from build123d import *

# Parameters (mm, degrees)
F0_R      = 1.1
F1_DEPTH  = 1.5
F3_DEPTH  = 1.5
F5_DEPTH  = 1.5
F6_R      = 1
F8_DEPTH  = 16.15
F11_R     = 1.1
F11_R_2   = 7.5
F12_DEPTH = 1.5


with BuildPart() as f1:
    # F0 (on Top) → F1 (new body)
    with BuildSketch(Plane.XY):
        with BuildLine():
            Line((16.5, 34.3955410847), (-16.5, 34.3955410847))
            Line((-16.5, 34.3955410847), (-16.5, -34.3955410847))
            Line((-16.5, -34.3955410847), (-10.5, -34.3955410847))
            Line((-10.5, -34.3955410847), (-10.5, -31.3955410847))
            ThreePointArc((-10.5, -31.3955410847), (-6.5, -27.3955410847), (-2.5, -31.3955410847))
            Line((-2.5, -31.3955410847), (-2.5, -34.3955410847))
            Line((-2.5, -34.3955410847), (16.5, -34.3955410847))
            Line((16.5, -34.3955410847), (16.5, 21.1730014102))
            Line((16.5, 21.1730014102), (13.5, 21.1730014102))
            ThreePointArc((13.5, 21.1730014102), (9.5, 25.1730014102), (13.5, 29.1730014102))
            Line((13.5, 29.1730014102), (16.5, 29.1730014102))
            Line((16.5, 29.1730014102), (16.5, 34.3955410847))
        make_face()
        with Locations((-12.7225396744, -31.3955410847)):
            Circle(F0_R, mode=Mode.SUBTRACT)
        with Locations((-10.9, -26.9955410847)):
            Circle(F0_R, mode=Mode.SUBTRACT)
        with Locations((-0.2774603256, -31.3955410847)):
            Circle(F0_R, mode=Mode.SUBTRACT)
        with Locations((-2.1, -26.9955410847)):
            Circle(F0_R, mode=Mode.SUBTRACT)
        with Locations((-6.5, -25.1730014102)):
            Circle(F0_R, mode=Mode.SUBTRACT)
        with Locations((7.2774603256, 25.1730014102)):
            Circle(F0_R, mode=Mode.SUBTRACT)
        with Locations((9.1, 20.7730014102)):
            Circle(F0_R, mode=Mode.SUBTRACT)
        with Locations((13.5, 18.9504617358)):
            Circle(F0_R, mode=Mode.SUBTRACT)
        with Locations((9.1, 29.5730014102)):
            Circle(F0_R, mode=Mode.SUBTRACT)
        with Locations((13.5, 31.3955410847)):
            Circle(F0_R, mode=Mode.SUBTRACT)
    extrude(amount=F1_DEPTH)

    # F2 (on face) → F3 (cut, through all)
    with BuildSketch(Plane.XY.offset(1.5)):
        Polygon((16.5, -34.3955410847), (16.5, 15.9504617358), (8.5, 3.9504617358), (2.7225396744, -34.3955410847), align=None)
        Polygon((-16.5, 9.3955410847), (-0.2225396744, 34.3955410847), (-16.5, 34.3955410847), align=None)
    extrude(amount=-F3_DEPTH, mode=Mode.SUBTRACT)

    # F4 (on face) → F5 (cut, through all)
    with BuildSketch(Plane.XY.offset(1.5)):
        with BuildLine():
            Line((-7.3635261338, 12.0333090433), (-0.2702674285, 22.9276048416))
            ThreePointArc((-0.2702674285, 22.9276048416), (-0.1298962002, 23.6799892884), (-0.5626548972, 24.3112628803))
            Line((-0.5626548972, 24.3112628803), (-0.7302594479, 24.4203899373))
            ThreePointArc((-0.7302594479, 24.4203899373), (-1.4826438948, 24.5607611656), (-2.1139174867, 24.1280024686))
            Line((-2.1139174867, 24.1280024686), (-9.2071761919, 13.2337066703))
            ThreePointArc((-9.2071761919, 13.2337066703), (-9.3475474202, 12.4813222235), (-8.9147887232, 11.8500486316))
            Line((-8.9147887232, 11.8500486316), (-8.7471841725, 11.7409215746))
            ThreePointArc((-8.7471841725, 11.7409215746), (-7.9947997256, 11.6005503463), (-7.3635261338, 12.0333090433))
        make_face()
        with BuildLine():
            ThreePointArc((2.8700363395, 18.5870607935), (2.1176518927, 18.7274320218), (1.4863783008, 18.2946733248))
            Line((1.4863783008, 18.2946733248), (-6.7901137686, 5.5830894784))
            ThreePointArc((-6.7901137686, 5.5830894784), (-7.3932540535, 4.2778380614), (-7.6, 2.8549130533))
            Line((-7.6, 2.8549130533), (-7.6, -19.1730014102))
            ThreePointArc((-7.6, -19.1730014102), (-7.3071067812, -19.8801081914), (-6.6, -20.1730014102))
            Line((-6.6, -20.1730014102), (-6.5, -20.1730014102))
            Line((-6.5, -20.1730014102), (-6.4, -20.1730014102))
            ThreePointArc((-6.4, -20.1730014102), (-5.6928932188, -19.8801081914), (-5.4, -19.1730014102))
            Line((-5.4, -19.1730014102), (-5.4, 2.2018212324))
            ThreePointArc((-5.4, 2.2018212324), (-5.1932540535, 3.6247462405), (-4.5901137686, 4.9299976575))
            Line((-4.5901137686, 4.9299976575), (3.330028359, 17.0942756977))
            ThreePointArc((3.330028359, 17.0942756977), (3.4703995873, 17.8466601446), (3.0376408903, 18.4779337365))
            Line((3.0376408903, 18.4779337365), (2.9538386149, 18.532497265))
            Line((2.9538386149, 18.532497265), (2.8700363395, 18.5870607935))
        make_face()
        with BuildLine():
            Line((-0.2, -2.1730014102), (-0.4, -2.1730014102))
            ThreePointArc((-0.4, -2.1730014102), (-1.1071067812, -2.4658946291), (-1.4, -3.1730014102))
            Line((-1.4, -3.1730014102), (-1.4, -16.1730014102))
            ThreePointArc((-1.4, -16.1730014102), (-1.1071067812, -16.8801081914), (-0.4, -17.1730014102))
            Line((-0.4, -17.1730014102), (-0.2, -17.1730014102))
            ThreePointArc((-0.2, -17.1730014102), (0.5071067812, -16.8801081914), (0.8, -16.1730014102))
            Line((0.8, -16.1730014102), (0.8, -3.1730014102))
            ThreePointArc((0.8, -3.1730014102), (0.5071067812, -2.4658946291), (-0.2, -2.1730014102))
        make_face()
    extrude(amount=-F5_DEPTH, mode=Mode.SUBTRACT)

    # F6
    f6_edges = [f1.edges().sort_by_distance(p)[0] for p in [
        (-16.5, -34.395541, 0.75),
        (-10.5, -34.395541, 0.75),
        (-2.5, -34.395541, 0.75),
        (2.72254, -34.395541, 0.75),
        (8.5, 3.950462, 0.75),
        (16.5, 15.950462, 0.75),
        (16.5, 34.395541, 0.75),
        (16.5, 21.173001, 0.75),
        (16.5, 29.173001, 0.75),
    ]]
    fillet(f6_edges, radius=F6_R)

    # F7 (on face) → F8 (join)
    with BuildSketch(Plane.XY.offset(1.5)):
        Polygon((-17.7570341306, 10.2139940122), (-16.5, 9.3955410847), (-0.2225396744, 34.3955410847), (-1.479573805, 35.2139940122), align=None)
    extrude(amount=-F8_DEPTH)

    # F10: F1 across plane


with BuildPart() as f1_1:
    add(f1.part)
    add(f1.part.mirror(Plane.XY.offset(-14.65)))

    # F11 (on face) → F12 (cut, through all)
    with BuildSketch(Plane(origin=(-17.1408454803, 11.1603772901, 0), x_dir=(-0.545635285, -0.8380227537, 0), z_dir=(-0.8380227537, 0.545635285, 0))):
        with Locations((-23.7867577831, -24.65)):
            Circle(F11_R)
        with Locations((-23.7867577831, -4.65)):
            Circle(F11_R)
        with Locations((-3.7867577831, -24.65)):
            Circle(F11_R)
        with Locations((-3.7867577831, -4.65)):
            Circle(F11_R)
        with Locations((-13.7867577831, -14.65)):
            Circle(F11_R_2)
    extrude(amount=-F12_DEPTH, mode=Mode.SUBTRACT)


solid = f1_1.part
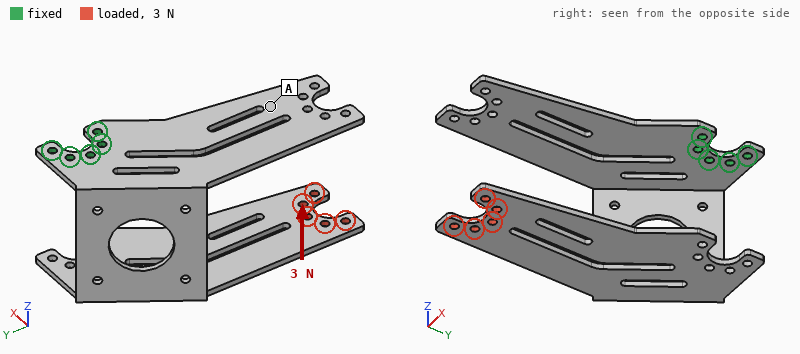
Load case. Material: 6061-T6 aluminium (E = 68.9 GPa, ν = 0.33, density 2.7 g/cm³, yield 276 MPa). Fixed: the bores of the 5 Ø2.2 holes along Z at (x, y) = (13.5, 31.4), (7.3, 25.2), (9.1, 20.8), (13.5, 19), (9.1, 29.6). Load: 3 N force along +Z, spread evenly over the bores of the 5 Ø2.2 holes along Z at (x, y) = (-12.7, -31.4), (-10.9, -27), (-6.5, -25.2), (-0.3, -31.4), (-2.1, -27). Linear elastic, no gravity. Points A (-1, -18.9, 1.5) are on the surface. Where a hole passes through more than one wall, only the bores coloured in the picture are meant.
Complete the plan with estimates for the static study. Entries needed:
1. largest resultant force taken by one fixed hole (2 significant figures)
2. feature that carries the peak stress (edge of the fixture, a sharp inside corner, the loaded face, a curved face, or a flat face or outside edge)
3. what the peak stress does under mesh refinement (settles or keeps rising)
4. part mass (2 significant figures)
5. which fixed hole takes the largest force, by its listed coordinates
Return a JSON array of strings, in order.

["15 N", "edge of the fixture", "keeps rising", "14 g", "(9.1, 29.6)"]
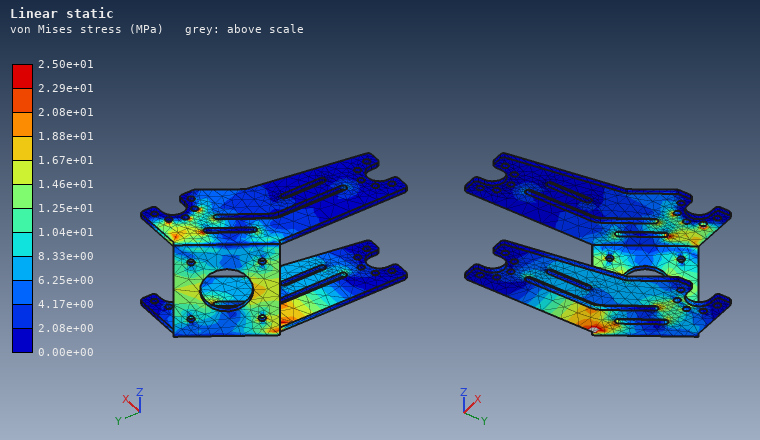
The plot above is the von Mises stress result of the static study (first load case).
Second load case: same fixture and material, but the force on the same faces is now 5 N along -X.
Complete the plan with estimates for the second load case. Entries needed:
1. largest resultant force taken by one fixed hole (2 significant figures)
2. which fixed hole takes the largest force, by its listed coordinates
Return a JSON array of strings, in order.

["19 N", "(7.3, 25.2)"]
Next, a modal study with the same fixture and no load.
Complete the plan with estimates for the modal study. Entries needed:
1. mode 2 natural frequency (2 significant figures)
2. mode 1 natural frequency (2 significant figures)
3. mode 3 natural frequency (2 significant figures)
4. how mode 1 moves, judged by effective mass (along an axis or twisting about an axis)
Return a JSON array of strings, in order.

["270 Hz", "210 Hz", "490 Hz", "along X"]
